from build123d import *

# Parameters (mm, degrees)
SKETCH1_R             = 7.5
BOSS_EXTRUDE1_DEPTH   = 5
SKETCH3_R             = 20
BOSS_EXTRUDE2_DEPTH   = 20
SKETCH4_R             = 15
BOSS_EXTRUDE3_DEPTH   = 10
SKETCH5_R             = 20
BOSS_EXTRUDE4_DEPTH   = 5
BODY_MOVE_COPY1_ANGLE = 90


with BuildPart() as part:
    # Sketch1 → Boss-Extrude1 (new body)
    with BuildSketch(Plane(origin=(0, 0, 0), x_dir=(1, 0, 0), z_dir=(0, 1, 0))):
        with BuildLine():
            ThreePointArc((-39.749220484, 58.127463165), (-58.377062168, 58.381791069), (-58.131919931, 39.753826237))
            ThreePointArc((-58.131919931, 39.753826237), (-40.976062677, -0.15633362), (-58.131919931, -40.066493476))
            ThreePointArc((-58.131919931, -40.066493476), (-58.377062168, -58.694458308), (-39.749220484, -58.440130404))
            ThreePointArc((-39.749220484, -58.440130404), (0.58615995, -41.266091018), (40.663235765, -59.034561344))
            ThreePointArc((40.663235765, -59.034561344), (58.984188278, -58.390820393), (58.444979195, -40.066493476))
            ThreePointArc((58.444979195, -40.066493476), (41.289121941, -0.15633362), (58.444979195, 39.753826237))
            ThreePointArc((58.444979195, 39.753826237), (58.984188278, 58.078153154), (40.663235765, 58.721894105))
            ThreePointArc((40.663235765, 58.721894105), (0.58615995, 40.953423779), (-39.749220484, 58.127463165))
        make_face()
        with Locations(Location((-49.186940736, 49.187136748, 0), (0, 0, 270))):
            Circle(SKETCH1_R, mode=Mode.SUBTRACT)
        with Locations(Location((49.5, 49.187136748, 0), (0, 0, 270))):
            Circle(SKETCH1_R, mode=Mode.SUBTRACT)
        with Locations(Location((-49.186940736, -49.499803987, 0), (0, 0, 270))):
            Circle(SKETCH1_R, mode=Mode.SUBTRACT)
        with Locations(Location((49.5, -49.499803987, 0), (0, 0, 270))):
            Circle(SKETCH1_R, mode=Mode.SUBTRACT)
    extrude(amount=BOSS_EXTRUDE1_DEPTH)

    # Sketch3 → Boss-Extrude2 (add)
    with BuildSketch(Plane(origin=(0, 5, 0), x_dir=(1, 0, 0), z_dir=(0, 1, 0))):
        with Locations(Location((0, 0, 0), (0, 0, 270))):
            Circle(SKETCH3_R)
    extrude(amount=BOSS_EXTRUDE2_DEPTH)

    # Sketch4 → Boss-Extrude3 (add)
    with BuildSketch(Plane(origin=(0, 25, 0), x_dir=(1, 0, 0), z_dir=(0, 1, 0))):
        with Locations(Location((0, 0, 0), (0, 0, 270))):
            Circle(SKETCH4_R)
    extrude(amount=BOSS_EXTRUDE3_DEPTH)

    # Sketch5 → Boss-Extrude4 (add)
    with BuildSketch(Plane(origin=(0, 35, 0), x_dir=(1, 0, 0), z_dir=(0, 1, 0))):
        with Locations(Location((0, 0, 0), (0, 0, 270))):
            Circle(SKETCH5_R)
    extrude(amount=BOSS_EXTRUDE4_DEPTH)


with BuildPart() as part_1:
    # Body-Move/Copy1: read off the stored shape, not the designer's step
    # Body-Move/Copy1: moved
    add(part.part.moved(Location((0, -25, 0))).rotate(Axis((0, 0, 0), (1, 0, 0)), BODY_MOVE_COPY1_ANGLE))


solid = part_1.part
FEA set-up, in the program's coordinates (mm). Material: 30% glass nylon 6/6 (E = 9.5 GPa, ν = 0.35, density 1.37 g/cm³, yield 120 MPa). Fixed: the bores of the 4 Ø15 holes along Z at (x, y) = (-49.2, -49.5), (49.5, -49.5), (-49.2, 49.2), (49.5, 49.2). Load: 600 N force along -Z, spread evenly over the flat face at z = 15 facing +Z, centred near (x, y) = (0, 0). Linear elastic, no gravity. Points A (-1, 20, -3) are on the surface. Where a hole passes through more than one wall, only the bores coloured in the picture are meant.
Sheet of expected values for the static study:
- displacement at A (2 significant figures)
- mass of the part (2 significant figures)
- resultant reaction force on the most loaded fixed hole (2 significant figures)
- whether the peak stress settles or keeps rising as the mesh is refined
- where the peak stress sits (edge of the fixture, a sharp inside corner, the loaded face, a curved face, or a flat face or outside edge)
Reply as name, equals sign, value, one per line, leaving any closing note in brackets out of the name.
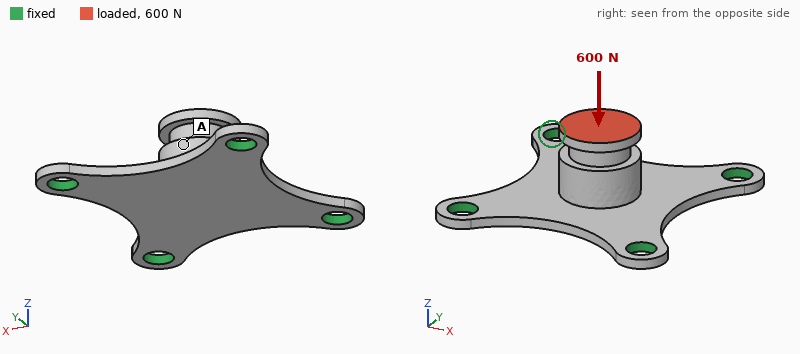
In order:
displacement at A = 0.34 mm
mass of the part = 120 g
resultant reaction force on the most loaded fixed hole = 160 N
whether the peak stress settles or keeps rising as the mesh is refined = keeps rising
where the peak stress sits = edge of the fixture
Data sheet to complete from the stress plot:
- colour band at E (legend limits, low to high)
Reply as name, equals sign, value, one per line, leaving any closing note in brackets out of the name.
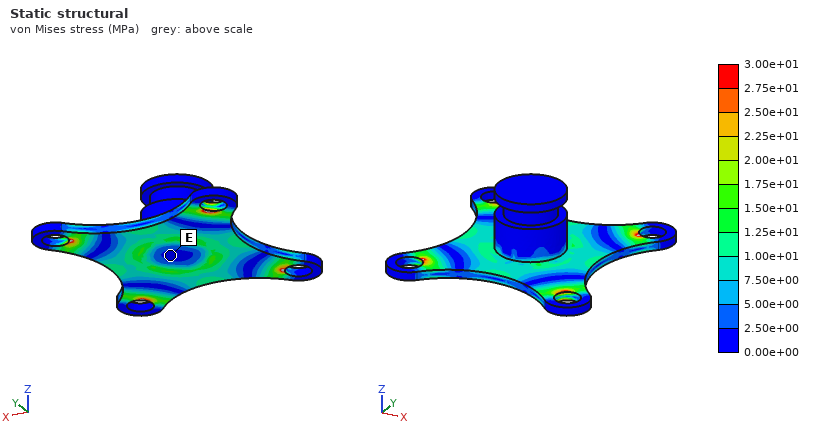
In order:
colour band at E = 0.00e+00 to 2.50e+00 MPa
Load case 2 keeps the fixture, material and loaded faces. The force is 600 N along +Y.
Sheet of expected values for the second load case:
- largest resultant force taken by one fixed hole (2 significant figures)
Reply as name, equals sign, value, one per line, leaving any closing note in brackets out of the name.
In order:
largest resultant force taken by one fixed hole = 240 N
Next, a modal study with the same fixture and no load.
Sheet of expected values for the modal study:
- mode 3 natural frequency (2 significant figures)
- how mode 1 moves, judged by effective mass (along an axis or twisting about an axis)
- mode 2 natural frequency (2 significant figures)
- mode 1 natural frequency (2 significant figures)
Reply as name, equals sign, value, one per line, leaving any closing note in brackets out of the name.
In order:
mode 3 natural frequency = 1100 Hz
how mode 1 moves, judged by effective mass = along Z
mode 2 natural frequency = 1100 Hz
mode 1 natural frequency = 740 Hz
